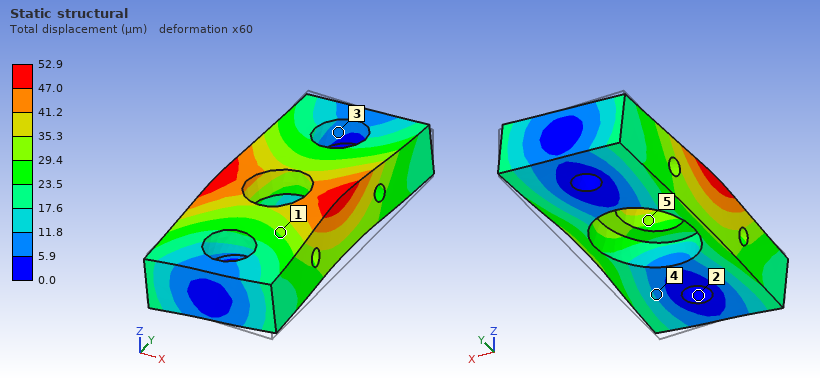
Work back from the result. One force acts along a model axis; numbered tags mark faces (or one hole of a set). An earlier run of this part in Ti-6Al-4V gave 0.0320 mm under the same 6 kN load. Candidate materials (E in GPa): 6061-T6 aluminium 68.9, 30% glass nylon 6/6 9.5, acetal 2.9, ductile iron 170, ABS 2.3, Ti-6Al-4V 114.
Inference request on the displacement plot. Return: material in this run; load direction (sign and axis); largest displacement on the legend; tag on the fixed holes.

6061-T6 aluminium
-X
52.9 µm
2
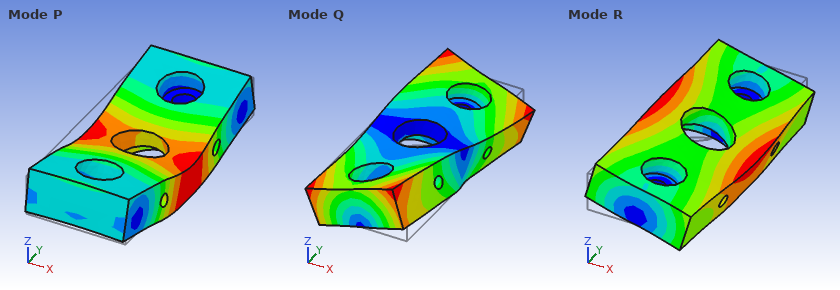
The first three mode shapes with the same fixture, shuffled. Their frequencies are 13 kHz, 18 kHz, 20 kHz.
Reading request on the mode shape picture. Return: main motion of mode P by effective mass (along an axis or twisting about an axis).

along Z
